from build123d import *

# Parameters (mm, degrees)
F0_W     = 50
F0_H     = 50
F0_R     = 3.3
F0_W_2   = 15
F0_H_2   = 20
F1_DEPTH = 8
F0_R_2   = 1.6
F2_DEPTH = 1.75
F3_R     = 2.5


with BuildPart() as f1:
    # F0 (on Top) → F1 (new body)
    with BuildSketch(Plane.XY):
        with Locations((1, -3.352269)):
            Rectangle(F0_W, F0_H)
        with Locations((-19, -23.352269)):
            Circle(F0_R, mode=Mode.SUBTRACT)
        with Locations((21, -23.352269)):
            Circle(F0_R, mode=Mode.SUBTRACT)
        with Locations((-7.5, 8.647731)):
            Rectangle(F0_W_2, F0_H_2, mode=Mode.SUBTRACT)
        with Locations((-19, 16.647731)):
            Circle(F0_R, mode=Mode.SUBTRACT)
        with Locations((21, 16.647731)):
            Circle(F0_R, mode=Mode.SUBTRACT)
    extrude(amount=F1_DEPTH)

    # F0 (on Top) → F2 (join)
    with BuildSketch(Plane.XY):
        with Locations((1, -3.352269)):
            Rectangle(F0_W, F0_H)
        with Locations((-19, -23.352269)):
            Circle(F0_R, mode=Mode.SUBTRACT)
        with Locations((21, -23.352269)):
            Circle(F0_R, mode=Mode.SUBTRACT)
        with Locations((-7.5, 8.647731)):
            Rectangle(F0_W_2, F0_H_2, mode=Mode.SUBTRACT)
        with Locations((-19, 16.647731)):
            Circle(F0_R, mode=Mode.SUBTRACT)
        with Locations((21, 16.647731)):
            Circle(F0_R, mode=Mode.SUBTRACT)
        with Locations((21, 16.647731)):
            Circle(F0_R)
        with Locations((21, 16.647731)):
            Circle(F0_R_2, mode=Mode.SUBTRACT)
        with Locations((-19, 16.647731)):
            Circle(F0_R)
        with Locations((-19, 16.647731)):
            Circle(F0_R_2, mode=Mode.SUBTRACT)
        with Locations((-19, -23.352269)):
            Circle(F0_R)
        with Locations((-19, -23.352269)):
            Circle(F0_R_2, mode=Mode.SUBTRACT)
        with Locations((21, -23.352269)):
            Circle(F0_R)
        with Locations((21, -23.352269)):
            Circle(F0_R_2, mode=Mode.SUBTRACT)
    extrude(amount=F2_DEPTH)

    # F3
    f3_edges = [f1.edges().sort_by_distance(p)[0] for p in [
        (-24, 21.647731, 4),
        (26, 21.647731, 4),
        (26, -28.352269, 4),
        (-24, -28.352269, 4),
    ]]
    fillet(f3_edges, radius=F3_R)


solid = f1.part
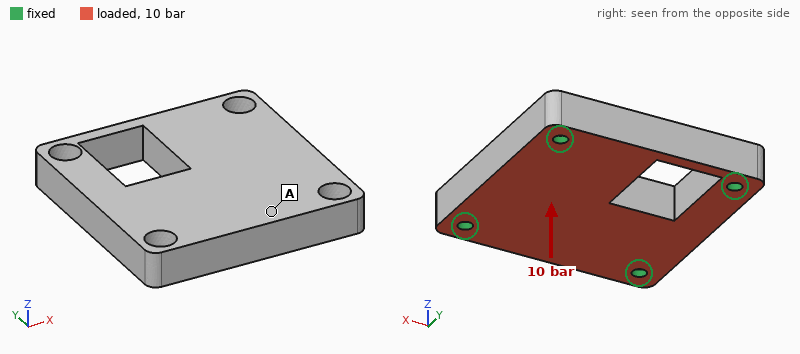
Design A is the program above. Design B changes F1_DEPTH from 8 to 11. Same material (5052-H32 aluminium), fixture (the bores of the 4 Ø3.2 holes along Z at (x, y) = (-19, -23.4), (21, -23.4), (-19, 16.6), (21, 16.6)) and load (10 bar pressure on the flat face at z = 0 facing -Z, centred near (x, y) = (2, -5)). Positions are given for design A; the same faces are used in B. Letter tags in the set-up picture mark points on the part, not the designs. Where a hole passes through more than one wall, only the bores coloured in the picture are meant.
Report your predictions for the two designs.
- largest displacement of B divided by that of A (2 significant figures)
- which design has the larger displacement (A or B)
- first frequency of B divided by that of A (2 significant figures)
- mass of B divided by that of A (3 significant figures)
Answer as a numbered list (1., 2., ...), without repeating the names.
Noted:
1. 0.55
2. A
3. 1.1
4. 1.37
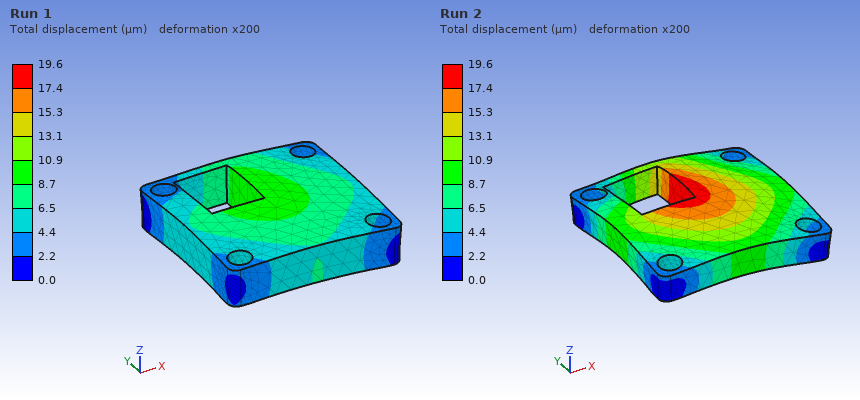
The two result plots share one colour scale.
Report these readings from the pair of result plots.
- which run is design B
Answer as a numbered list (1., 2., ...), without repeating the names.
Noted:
1. Run 1
